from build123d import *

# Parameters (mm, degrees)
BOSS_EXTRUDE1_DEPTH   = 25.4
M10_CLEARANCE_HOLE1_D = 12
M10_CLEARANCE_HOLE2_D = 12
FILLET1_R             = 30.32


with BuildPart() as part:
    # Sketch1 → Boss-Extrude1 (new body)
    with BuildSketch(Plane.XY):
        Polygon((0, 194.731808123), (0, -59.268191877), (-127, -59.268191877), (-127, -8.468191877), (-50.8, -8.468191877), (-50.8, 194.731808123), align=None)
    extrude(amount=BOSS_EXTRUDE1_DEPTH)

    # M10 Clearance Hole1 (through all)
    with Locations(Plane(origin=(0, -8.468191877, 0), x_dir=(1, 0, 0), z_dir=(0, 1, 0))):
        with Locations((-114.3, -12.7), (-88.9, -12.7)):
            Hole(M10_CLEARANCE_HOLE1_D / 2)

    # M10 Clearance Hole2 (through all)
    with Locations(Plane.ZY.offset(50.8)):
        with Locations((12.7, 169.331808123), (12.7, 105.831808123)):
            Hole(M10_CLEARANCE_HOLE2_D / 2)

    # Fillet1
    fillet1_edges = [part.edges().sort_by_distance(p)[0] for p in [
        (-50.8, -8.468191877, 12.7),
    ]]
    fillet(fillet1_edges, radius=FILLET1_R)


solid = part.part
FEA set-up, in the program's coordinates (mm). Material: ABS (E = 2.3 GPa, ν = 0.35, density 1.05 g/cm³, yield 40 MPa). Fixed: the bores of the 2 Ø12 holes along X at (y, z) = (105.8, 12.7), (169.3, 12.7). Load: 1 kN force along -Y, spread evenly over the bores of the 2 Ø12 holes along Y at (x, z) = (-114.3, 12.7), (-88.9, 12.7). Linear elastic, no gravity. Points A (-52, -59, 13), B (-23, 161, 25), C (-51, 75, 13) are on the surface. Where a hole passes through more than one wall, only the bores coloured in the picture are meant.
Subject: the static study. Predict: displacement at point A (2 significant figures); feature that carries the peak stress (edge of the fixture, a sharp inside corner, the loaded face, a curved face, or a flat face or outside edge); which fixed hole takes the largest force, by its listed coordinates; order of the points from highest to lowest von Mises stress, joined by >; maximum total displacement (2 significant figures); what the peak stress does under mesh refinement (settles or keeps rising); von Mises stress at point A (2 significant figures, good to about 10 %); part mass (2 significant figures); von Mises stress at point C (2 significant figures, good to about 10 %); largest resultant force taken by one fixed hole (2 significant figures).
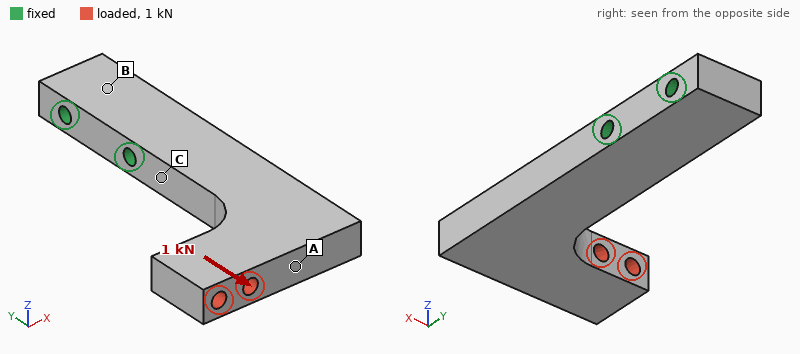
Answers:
1.5 mm
edge of the fixture
(105.8, 12.7)
C > A > B
2.2 mm
keeps rising
2.8 MPa
430 g
7.8 MPa
980 N
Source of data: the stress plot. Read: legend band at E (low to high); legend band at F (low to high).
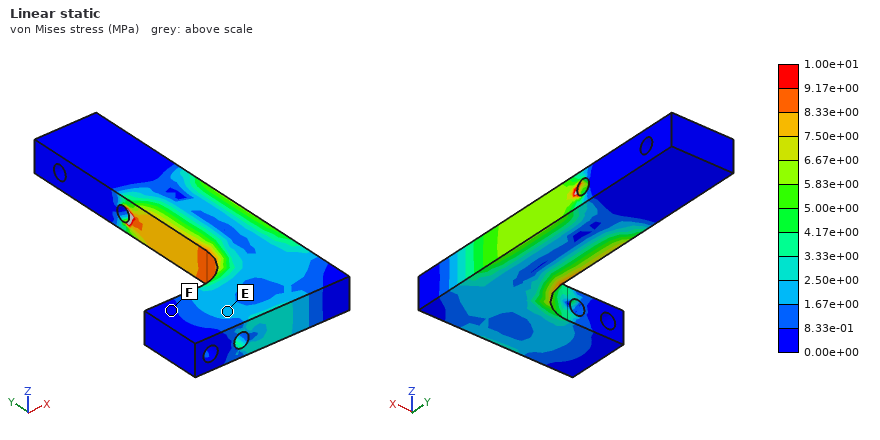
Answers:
1.67e+00 to 2.50e+00 MPa
0.00e+00 to 8.33e-01 MPa
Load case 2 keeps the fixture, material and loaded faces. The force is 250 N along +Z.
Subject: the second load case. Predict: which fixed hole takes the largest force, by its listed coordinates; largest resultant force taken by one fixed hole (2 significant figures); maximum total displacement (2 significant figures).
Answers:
(105.8, 12.7)
370 N
3.4 mm
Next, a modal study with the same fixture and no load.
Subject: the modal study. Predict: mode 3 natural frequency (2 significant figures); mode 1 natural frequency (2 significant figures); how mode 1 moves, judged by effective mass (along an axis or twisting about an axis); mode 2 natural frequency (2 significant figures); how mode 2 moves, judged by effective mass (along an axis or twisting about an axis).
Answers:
380 Hz
140 Hz
along Z
270 Hz
along X
